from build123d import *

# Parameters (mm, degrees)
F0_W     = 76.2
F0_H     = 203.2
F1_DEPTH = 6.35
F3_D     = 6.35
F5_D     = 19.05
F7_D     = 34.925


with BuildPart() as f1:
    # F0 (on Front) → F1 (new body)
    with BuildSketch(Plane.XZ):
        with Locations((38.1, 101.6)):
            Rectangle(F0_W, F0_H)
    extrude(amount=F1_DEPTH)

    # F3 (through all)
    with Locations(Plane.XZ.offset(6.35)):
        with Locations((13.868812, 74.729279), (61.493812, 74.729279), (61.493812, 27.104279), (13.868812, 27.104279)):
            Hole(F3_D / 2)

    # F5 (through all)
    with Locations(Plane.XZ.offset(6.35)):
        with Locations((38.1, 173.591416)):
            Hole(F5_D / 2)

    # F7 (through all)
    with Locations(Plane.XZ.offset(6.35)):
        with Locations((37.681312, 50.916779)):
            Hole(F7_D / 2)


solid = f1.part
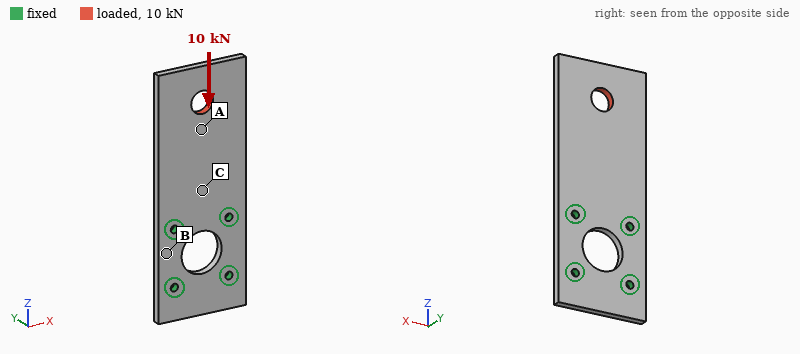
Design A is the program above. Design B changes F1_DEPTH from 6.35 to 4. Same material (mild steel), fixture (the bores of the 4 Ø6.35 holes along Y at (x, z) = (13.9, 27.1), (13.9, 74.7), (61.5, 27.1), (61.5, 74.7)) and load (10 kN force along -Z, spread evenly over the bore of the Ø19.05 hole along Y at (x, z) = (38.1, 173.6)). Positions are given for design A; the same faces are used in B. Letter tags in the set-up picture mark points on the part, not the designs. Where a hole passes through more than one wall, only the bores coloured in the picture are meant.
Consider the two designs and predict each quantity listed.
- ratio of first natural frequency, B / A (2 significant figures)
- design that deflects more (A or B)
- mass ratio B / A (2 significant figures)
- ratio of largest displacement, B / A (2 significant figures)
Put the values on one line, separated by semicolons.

0.64; B; 0.63; 1.6
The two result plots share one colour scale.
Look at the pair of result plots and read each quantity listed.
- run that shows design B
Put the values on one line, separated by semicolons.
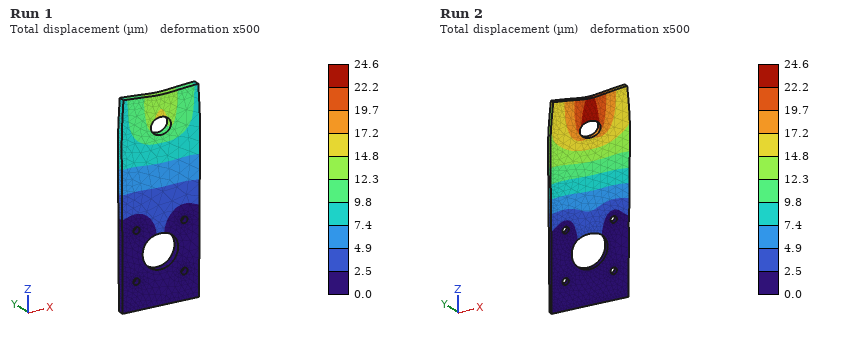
Run 2
